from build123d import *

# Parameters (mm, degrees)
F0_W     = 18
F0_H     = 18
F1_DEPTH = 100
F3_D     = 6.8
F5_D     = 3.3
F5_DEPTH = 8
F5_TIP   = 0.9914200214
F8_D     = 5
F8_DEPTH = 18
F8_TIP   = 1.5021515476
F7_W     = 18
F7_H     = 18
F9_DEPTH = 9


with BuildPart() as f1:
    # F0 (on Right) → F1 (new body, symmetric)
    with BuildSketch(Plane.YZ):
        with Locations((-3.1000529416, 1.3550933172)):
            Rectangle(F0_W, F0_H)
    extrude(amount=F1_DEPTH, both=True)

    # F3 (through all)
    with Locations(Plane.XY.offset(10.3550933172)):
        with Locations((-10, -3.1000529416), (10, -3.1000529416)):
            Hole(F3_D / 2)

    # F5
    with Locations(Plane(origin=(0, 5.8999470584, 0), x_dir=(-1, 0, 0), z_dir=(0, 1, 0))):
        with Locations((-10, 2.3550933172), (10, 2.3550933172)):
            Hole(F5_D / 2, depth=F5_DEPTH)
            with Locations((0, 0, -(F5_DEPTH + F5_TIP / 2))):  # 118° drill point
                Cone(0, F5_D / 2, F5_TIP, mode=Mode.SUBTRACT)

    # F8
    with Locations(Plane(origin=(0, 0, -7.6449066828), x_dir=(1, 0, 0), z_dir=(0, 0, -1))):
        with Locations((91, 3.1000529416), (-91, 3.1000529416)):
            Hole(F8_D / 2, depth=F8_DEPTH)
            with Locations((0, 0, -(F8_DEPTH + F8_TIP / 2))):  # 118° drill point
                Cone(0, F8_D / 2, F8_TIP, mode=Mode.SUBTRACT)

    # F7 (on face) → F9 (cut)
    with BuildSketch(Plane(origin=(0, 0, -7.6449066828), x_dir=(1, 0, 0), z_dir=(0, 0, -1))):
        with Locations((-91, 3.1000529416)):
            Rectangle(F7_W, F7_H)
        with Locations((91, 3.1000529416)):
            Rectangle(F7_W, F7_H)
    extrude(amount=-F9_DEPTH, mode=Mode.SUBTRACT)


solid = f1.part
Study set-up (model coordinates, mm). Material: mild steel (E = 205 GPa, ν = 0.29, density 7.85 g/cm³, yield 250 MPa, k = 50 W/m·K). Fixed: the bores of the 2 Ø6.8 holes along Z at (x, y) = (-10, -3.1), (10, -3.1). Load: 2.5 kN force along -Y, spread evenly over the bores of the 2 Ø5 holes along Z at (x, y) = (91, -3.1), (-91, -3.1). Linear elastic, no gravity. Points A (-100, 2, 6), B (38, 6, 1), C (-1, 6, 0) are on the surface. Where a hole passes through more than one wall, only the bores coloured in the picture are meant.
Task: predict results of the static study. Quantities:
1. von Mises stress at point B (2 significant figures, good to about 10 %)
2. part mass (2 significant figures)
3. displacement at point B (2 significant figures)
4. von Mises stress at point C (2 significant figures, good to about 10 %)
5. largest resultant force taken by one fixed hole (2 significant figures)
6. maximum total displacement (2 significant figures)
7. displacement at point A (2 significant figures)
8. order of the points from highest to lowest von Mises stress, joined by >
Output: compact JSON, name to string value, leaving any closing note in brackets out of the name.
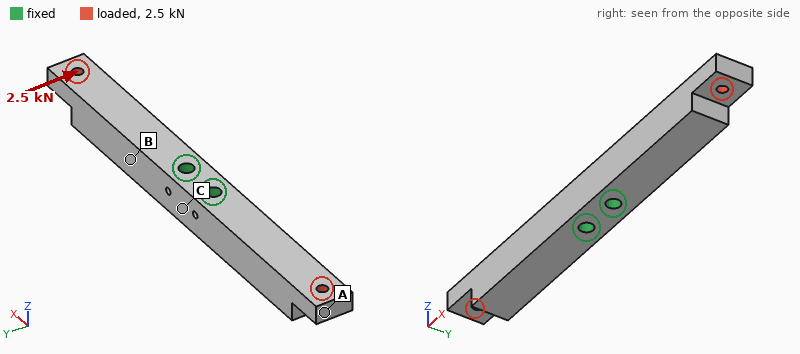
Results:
{"von Mises stress at point B": "68 MPa", "part mass": "450 g", "displacement at point B": "0.030 mm", "von Mises stress at point C": "36 MPa", "largest resultant force taken by one fixed hole": "1.3 kN", "maximum total displacement": "0.17 mm", "displacement at point A": "0.17 mm", "order of the points from highest to lowest von Mises stress, joined by >": "B > C > A"}
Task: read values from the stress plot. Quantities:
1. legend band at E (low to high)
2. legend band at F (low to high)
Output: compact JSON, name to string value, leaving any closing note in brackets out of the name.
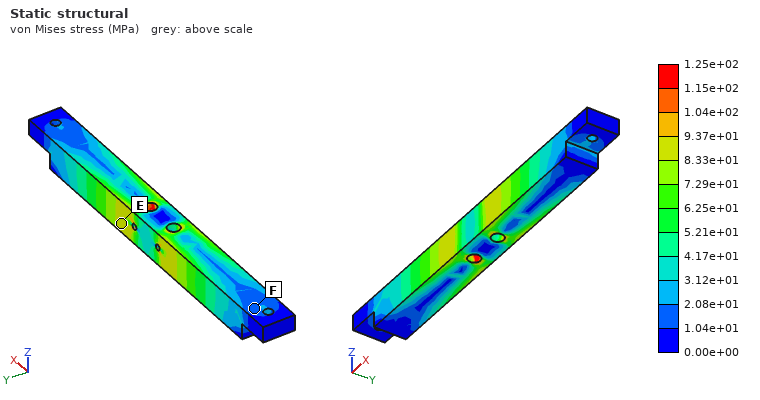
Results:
{"legend band at E": "8.33e+01 to 9.37e+01 MPa", "legend band at F": "1.04e+01 to 2.08e+01 MPa"}
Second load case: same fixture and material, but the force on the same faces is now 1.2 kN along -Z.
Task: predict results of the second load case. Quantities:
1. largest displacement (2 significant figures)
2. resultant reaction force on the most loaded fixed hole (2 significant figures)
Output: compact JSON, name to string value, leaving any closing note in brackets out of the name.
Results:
{"largest displacement": "74 µm", "resultant reaction force on the most loaded fixed hole": "600 N"}
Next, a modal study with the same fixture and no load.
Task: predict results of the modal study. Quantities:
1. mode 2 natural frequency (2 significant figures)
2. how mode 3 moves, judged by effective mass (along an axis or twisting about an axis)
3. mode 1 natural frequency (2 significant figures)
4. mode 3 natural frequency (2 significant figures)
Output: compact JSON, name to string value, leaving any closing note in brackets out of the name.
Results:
{"mode 2 natural frequency": "2000 Hz", "how mode 3 moves, judged by effective mass": "twisting about Y", "mode 1 natural frequency": "2000 Hz", "mode 3 natural frequency": "2200 Hz"}
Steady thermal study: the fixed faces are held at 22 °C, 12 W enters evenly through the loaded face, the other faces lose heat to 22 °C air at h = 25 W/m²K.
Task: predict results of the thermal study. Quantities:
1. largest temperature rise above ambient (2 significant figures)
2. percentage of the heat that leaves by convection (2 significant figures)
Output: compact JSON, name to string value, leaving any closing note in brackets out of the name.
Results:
{"largest temperature rise above ambient": "29 K", "percentage of the heat that leaves by convection": "33 %"}
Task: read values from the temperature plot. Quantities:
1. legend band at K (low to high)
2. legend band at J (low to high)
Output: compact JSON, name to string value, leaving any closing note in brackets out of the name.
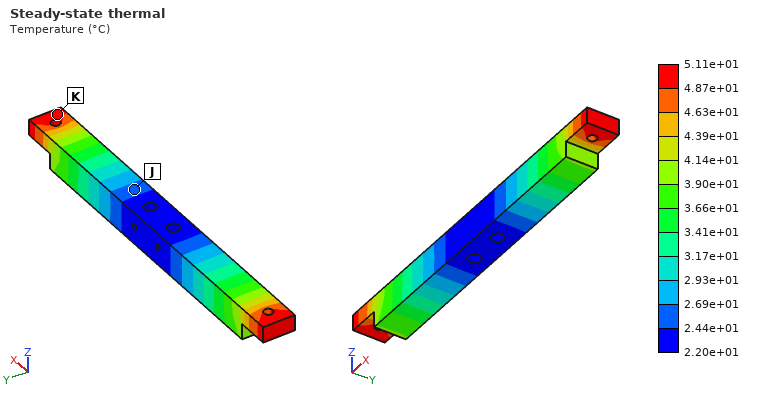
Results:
{"legend band at K": "4.87e+01 to 5.11e+01 °C", "legend band at J": "2.44e+01 to 2.69e+01 °C"}
